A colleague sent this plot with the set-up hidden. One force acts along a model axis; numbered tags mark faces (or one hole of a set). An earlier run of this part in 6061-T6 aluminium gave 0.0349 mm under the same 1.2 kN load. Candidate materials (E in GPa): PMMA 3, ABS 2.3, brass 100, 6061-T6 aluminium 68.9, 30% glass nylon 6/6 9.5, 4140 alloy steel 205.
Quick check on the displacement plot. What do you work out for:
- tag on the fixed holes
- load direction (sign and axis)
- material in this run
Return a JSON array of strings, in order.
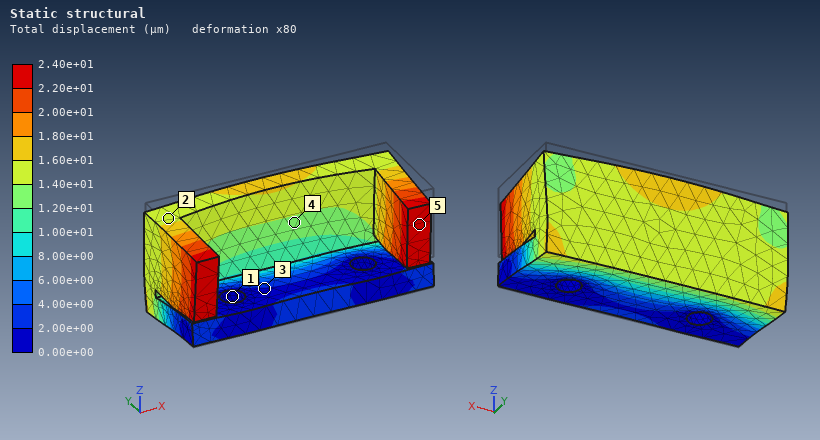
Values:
["1", "-Z", "brass"]
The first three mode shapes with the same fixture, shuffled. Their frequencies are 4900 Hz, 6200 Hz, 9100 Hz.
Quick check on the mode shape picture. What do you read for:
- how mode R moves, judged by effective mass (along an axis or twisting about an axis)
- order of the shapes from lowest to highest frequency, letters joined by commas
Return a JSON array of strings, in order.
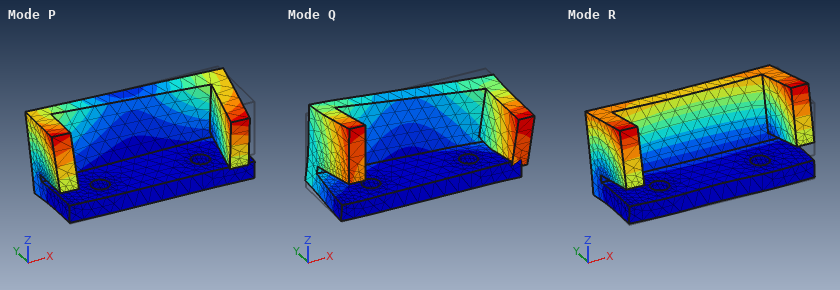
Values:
["along Y", "R, P, Q"]
